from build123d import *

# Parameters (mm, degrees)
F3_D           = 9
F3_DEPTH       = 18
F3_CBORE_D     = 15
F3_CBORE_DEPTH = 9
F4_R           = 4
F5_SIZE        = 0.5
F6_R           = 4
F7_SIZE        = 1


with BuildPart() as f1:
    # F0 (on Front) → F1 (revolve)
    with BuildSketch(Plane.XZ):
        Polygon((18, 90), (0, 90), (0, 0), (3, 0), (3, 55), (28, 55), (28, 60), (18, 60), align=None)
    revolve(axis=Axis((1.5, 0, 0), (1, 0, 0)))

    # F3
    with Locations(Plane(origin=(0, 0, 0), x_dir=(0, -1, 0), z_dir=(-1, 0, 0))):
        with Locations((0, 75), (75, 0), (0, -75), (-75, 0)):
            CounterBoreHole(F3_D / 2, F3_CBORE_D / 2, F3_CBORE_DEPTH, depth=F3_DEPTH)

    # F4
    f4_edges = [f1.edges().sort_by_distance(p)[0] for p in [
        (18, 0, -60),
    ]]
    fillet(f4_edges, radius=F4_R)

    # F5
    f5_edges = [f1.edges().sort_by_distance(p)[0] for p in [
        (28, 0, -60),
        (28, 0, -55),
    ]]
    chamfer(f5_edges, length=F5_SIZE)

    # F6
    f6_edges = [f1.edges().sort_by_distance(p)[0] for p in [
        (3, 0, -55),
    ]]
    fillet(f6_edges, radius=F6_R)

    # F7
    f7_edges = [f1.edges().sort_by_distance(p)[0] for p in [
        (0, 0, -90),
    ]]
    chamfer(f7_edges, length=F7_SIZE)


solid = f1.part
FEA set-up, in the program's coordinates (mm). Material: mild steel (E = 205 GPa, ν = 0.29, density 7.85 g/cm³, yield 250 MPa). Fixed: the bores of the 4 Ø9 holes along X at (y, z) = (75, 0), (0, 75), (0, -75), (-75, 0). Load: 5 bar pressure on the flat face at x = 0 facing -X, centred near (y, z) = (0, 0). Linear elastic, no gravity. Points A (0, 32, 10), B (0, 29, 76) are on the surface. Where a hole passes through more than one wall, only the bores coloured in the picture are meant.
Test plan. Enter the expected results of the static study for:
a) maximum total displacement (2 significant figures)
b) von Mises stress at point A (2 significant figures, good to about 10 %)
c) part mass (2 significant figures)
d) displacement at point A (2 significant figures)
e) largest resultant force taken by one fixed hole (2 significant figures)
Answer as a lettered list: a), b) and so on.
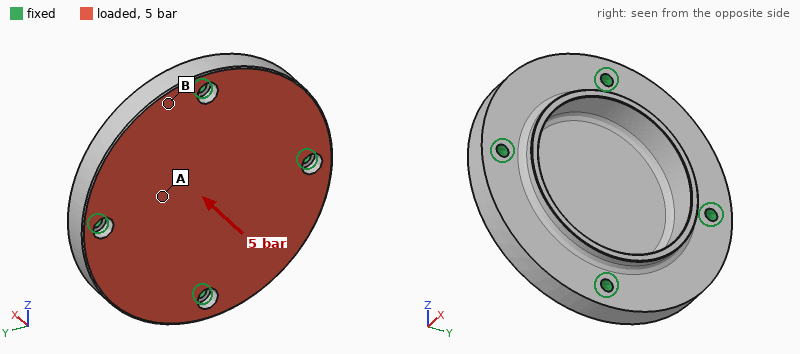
a) 0.14 mm
b) 37 MPa
c) 2.6 kg
d) 0.057 mm
e) 3.4 kN
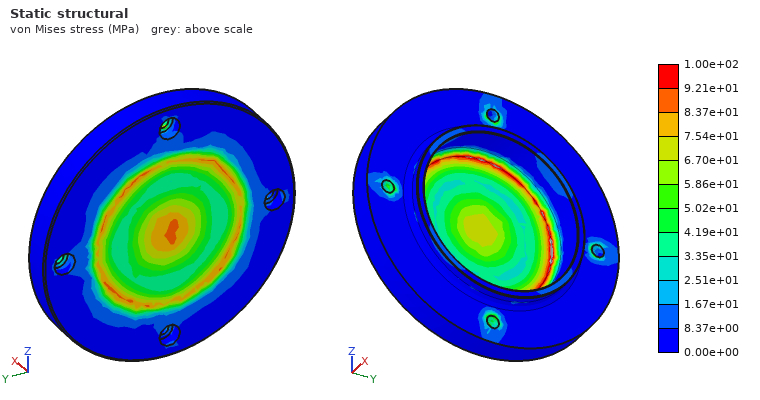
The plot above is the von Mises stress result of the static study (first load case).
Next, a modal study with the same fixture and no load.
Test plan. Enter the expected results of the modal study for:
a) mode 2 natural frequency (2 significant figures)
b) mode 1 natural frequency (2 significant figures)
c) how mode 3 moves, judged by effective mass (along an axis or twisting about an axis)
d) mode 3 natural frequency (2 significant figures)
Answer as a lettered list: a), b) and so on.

a) 4000 Hz
b) 2500 Hz
c) twisting about Y
d) 4800 Hz
